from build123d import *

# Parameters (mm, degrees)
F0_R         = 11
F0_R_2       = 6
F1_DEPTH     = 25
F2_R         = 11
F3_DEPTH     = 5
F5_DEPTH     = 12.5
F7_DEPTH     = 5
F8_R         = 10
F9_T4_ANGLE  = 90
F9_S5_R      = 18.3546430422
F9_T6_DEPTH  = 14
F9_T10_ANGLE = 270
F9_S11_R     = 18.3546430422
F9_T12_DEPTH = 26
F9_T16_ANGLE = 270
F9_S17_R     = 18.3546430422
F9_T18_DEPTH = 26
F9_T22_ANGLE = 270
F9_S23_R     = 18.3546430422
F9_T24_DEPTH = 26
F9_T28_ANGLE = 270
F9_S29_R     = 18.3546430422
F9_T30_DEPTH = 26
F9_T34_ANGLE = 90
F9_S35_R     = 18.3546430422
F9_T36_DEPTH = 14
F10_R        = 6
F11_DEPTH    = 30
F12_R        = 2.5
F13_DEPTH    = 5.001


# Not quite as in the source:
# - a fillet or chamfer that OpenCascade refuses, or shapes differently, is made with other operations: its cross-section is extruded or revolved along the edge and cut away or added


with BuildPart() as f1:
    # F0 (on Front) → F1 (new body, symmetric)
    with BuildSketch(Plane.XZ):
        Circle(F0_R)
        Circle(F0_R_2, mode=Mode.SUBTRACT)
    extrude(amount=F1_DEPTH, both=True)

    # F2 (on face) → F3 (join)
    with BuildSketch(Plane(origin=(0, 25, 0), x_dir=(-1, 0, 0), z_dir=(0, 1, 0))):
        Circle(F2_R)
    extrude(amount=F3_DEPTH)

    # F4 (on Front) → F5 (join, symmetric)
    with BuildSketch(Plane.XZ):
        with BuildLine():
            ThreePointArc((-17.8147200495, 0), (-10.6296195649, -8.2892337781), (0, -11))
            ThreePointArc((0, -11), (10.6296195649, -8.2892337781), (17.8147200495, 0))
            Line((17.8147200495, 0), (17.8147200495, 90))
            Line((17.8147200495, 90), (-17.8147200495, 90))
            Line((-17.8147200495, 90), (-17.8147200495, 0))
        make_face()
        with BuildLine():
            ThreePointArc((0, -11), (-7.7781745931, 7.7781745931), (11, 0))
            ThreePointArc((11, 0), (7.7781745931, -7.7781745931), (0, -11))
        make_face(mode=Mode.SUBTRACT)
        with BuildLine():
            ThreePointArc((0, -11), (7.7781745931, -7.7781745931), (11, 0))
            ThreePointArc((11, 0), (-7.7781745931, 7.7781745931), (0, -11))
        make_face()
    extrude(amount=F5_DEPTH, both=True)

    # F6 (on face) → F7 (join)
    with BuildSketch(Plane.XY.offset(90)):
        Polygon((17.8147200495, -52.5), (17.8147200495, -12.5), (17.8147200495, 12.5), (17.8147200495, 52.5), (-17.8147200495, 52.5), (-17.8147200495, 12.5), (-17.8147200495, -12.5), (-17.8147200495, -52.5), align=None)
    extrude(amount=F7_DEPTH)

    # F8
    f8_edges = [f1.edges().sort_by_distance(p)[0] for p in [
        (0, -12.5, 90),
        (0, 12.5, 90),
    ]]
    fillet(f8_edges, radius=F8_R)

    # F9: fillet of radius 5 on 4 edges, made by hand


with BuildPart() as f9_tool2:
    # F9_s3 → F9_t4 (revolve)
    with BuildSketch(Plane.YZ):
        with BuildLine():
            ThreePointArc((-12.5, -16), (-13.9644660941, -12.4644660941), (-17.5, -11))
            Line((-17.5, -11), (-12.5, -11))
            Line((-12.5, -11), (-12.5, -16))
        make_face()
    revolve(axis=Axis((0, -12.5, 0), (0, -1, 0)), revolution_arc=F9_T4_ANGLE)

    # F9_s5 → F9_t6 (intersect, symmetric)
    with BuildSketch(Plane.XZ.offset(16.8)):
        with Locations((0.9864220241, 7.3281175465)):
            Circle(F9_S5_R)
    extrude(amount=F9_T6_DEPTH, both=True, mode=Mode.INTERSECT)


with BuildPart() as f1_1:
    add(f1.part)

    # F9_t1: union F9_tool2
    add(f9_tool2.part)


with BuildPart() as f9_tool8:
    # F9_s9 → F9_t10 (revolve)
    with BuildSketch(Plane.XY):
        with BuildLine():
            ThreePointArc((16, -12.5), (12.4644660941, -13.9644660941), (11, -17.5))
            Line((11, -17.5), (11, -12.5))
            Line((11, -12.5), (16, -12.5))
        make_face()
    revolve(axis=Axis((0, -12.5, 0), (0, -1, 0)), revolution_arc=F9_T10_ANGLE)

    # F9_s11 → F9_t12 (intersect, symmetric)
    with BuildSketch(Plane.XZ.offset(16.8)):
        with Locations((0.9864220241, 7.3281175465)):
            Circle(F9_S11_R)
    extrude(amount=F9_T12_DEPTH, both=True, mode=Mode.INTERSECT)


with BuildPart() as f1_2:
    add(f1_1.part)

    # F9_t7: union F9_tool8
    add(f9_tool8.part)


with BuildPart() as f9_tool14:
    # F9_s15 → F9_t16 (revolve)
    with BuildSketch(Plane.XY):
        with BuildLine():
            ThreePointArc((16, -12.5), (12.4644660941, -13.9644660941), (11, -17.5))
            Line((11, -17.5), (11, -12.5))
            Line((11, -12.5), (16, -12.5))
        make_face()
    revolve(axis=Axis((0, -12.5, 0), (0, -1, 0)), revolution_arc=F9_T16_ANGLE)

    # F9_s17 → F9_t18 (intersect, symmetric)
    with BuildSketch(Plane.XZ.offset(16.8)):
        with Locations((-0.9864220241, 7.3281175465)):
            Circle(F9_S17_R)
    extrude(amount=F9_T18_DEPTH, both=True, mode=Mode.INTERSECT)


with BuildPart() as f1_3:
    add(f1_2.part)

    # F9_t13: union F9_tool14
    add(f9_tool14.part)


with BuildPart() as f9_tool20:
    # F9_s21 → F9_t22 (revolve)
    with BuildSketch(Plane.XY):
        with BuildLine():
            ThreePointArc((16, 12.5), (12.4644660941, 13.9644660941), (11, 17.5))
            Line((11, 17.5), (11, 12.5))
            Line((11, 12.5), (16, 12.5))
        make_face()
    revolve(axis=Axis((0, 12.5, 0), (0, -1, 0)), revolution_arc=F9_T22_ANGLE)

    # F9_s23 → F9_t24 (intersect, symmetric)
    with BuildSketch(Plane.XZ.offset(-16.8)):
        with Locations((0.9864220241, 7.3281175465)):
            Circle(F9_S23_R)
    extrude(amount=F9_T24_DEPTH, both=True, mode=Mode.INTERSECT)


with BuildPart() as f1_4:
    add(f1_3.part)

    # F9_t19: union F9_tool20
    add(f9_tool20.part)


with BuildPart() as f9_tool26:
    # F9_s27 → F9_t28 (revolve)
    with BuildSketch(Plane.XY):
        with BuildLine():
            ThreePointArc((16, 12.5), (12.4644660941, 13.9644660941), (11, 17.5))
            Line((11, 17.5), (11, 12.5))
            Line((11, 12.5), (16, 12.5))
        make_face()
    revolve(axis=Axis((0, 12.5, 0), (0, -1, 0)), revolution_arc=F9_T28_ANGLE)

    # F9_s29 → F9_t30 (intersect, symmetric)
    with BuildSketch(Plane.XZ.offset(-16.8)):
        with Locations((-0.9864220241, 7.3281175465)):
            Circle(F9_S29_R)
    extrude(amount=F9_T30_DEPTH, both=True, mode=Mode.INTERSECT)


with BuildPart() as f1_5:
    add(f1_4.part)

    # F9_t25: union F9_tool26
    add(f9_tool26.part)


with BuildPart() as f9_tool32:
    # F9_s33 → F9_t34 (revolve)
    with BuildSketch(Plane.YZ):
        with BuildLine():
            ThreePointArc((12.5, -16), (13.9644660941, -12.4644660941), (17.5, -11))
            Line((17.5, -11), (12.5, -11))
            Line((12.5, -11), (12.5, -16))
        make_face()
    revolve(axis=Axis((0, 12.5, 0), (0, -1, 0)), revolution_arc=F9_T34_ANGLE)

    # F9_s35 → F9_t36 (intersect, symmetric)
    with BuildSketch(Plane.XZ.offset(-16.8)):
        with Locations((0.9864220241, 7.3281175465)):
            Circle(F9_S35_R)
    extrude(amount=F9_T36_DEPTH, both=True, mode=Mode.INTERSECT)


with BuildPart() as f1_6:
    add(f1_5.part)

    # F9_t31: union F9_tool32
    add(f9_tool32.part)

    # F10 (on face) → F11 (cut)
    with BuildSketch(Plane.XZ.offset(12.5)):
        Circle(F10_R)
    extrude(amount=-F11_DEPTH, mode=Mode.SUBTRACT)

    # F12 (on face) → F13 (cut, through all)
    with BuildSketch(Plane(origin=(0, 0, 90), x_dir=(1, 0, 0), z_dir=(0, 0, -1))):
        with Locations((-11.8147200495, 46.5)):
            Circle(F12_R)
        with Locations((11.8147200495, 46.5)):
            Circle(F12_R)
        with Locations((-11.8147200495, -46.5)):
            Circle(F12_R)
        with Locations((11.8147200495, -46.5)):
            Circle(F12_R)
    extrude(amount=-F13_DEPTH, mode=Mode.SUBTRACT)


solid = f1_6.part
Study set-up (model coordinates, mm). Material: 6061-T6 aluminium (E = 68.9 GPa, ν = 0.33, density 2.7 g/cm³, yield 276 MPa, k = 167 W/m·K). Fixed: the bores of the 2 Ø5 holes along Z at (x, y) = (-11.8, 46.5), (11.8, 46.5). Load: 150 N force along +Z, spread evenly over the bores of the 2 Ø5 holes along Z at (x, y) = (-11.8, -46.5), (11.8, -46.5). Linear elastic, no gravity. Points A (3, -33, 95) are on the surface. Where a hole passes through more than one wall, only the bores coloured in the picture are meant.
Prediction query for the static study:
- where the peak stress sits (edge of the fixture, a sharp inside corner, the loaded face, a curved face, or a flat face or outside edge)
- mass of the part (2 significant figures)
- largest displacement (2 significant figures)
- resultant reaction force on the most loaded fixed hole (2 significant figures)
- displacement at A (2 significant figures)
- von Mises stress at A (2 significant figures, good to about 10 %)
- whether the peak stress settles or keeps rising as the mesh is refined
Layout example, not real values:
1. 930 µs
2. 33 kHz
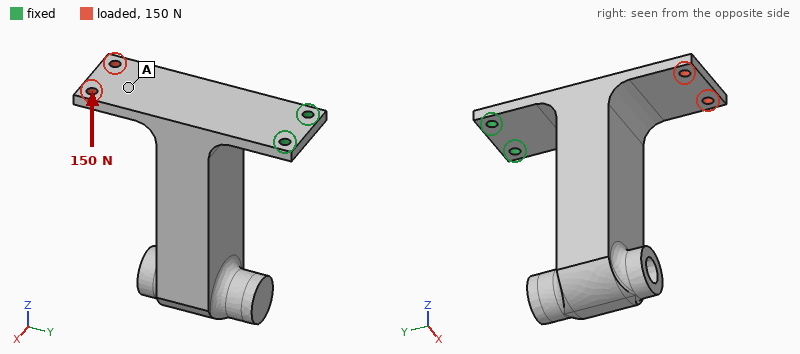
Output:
1. edge of the fixture
2. 310 g
3. 1.5 mm
4. 76 N
5. 0.88 mm
6. 12 MPa
7. keeps rising
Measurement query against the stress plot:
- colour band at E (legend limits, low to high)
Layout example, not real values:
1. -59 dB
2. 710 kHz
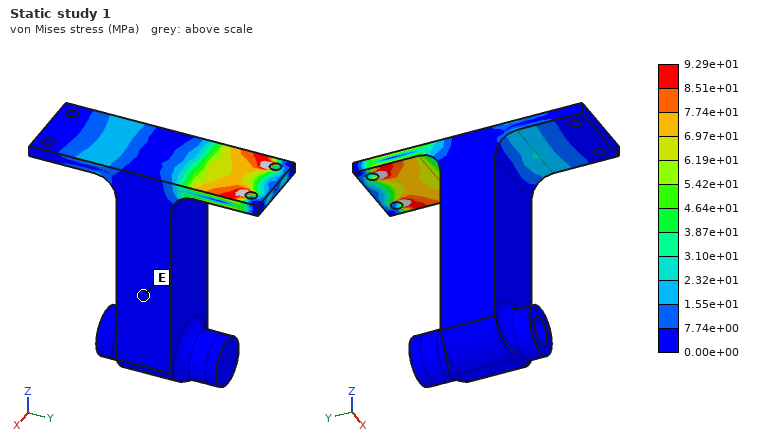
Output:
1. 0.00e+00 to 7.74e+00 MPa
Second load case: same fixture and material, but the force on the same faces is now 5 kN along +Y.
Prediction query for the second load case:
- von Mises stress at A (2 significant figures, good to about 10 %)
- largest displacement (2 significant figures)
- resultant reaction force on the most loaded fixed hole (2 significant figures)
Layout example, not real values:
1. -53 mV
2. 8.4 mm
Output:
1. 23 MPa
2. 0.11 mm
3. 2.5 kN
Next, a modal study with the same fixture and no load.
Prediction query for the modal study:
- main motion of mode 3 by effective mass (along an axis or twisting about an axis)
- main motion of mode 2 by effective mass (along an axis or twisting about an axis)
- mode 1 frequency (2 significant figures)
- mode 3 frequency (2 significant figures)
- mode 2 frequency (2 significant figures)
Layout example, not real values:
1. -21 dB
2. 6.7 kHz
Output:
1. along Z
2. along X
3. 130 Hz
4. 1000 Hz
5. 240 Hz
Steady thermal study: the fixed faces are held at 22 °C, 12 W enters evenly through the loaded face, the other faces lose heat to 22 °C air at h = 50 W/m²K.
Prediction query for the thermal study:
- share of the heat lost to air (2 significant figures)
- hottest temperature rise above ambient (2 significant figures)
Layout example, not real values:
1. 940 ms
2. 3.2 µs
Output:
1. 60 %
2. 21 K
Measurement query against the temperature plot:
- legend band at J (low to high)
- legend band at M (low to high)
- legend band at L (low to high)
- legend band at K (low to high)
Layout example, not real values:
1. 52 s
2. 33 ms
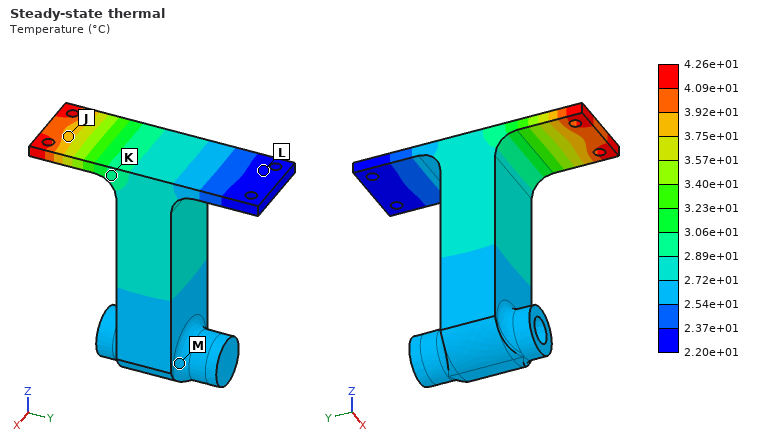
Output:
1. 3.75e+01 to 3.92e+01 °C
2. 2.54e+01 to 2.72e+01 °C
3. 2.20e+01 to 2.37e+01 °C
4. 2.89e+01 to 3.06e+01 °C
